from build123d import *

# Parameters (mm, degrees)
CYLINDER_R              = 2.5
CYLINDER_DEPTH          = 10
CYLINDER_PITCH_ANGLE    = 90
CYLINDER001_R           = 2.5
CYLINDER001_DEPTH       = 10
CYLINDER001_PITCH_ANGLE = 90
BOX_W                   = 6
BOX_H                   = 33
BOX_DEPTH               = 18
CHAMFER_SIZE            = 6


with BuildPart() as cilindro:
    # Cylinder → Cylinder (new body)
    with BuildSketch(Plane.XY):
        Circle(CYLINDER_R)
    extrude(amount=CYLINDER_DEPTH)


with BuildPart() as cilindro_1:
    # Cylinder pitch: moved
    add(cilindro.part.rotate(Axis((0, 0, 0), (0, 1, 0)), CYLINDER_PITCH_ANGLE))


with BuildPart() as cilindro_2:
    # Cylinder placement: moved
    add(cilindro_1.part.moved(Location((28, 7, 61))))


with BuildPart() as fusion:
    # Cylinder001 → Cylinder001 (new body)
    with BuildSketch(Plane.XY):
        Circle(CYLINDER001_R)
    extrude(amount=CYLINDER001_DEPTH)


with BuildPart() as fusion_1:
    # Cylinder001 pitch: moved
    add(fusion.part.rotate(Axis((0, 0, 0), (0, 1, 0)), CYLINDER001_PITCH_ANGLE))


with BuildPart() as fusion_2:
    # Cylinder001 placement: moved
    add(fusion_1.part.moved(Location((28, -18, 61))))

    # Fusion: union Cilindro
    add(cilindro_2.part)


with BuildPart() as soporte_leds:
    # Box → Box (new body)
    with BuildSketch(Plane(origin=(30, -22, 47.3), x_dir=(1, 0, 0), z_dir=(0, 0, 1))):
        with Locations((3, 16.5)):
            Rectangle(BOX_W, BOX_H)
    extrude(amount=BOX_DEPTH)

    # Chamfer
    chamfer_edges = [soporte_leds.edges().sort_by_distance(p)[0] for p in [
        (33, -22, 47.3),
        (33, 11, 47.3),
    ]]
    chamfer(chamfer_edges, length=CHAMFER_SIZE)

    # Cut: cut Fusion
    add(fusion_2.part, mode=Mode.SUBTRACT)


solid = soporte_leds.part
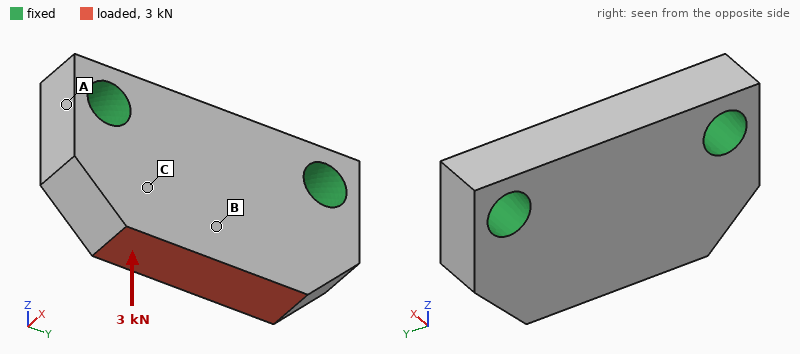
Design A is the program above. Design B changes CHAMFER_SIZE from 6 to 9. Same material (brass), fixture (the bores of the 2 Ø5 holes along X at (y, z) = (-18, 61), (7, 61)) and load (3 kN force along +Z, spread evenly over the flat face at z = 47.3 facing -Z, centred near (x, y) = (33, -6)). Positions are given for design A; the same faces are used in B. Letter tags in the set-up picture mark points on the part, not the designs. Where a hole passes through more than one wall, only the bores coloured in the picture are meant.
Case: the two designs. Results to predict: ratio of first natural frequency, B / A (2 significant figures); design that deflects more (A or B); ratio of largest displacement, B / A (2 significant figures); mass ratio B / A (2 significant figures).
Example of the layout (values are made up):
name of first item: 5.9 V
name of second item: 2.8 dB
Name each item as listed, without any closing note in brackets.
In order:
ratio of first natural frequency, B / A: 1.0
design that deflects more: B
ratio of largest displacement, B / A: 1.2
mass ratio B / A: 0.91
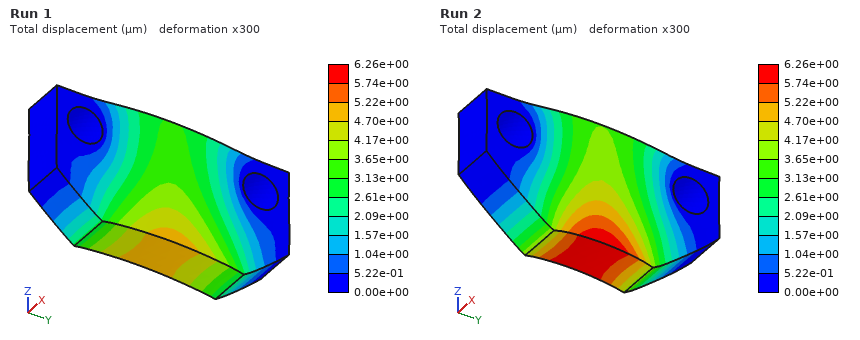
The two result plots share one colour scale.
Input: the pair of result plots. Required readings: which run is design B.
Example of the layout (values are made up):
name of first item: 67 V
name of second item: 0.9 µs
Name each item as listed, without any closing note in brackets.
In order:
which run is design B: Run 2
